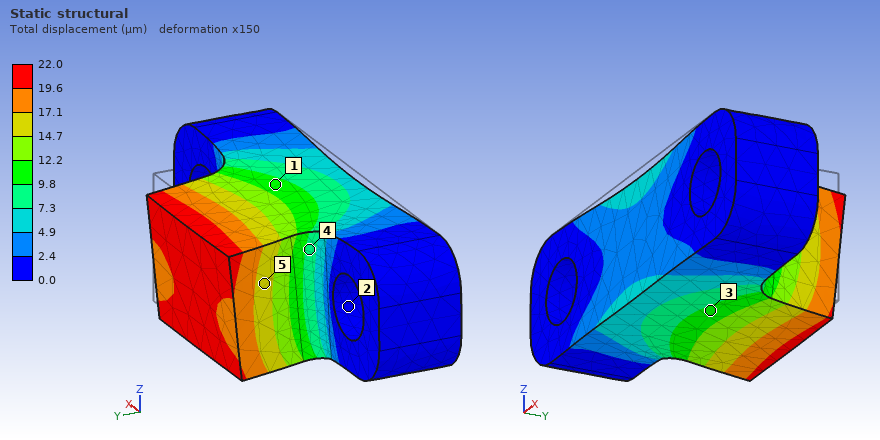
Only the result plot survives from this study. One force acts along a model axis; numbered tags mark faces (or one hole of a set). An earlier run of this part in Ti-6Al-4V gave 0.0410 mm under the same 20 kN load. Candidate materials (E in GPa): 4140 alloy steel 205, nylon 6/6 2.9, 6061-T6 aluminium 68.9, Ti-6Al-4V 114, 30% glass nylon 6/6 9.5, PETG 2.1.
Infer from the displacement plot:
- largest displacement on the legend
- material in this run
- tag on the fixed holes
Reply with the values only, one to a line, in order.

22.0 µm
4140 alloy steel
2
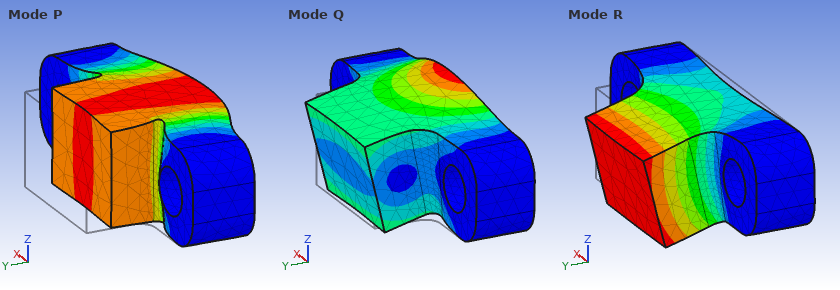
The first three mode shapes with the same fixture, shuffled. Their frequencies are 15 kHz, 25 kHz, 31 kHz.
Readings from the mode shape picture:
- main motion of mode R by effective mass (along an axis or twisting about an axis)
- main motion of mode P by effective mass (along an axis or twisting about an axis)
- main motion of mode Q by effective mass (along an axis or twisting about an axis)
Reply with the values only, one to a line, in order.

along Z
along Y
along Z
